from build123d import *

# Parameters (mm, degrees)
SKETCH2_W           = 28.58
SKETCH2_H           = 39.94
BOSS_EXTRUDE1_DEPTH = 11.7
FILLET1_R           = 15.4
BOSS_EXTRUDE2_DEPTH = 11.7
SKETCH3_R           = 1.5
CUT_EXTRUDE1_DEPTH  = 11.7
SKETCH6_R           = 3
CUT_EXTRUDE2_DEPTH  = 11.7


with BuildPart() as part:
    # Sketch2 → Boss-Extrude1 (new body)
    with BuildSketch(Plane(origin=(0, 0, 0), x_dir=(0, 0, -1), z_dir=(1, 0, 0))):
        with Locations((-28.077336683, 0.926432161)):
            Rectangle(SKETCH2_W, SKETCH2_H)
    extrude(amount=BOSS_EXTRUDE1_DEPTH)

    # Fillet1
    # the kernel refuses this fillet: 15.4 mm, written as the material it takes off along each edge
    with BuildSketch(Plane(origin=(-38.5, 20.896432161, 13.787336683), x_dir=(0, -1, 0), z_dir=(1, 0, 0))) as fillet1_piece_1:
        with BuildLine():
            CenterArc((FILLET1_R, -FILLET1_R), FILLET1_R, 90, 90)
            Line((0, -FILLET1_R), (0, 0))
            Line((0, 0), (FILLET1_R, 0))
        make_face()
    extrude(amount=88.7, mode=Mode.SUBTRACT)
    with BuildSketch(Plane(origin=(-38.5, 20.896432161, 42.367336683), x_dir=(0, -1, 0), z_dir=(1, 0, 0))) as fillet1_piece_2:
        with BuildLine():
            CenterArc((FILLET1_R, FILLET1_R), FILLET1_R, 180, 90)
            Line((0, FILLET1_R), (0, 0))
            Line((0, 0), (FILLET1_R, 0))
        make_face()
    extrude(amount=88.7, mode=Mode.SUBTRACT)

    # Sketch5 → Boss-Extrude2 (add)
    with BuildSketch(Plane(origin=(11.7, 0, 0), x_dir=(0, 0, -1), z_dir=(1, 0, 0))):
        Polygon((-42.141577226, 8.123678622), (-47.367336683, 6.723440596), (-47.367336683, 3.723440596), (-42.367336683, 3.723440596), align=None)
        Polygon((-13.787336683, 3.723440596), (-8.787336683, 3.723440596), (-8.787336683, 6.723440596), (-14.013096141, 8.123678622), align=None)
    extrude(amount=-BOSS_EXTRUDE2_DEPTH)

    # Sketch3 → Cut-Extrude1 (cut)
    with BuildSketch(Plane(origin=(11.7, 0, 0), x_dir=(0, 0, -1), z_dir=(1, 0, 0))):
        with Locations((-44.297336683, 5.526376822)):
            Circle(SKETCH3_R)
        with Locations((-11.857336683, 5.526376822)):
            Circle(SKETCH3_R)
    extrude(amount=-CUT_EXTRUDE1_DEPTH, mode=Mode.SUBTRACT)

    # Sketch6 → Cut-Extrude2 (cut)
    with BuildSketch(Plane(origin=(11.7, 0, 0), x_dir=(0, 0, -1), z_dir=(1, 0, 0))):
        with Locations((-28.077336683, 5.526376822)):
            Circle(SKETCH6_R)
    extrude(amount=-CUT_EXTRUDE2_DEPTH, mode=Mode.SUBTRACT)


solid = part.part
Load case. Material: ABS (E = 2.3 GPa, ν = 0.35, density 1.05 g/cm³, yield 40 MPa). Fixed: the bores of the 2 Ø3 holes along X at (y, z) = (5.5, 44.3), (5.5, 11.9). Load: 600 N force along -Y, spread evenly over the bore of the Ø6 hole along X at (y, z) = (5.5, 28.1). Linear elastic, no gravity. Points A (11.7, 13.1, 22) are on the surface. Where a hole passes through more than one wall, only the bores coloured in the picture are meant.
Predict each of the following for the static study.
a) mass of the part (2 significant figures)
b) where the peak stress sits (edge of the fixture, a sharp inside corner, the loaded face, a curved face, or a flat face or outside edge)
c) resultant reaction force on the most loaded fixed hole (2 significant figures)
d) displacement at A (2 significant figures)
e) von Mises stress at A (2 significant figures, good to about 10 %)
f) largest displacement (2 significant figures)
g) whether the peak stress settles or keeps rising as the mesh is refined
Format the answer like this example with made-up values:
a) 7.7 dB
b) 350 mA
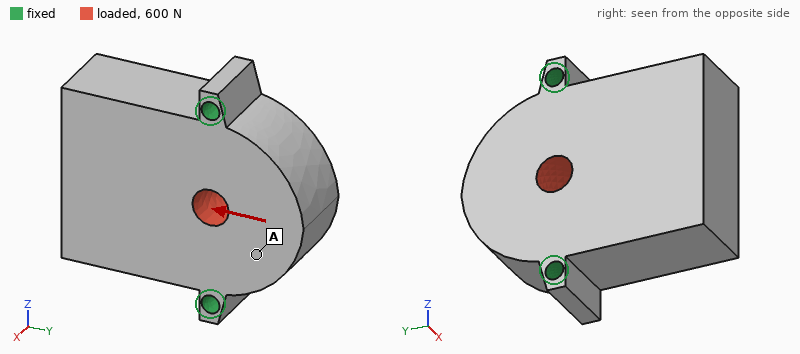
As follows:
a) 13 g
b) edge of the fixture
c) 300 N
d) 31 µm
e) 2.2 MPa
f) 40 µm
g) keeps rising
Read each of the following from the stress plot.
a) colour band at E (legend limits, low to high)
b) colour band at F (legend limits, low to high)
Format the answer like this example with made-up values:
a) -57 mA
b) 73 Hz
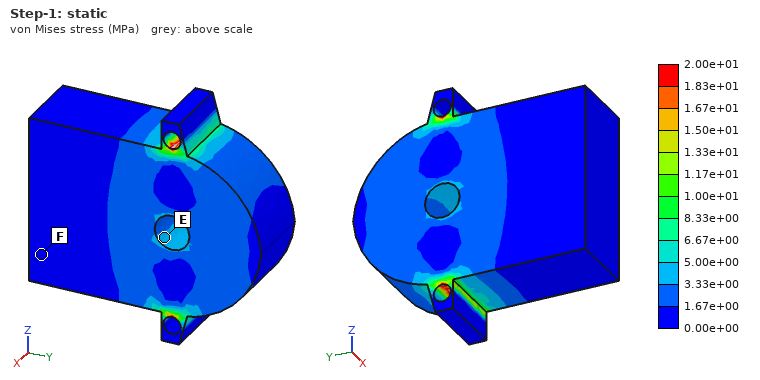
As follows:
a) 3.33e+00 to 5.00e+00 MPa
b) 0.00e+00 to 1.67e+00 MPa
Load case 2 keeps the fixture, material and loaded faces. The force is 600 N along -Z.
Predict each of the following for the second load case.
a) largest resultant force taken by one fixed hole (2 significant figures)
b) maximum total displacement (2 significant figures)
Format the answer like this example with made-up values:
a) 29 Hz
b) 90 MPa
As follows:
a) 300 N
b) 20 µm
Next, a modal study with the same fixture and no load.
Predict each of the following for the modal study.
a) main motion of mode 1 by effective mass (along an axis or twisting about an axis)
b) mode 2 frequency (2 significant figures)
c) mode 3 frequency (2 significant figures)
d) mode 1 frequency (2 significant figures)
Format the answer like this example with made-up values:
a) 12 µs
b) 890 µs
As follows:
a) along X
b) 5600 Hz
c) 5800 Hz
d) 2000 Hz
